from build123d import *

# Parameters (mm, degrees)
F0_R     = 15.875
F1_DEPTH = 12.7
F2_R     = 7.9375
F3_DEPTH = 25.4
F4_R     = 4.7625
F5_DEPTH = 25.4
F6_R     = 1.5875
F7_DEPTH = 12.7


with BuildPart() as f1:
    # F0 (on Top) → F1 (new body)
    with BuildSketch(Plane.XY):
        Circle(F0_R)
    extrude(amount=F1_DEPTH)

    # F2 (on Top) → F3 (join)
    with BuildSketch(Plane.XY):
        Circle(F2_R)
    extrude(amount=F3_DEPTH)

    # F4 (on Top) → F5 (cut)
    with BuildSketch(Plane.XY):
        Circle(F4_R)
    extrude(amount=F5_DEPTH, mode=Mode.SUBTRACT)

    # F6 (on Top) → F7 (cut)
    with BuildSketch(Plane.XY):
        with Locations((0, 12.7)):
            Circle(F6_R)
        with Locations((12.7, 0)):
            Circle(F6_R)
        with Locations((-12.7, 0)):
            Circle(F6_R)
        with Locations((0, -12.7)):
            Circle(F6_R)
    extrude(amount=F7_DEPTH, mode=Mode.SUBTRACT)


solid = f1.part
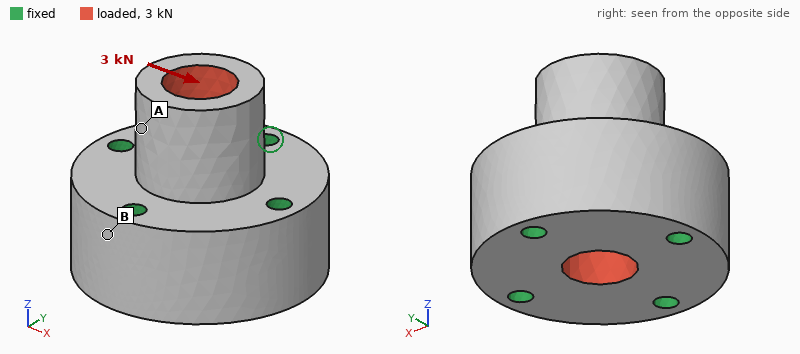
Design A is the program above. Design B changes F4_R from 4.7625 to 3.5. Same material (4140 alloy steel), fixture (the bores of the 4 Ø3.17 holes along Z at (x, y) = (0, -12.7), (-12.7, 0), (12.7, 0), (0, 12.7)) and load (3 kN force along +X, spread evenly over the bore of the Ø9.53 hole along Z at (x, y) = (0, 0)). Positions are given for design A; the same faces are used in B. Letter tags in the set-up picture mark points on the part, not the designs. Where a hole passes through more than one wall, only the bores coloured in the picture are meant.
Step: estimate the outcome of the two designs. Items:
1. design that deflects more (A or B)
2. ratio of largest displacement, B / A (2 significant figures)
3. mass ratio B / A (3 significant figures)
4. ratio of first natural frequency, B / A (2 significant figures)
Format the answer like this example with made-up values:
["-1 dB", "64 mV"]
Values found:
["A", "0.83", "1.08", "0.98"]
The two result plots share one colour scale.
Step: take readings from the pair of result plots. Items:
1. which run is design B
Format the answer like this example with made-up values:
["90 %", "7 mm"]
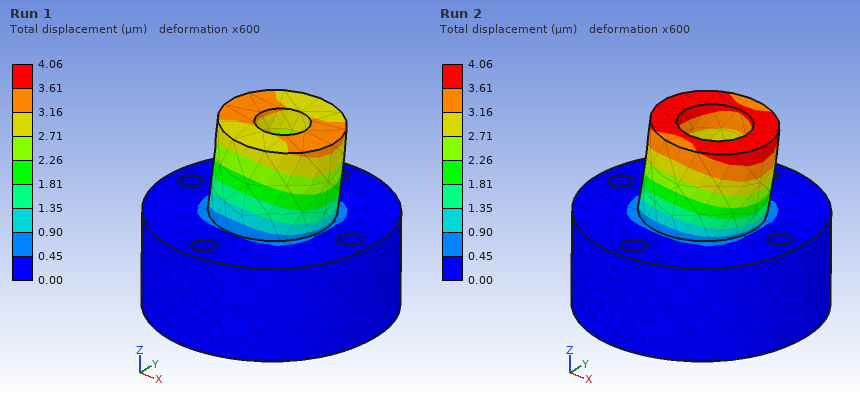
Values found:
["Run 1"]
